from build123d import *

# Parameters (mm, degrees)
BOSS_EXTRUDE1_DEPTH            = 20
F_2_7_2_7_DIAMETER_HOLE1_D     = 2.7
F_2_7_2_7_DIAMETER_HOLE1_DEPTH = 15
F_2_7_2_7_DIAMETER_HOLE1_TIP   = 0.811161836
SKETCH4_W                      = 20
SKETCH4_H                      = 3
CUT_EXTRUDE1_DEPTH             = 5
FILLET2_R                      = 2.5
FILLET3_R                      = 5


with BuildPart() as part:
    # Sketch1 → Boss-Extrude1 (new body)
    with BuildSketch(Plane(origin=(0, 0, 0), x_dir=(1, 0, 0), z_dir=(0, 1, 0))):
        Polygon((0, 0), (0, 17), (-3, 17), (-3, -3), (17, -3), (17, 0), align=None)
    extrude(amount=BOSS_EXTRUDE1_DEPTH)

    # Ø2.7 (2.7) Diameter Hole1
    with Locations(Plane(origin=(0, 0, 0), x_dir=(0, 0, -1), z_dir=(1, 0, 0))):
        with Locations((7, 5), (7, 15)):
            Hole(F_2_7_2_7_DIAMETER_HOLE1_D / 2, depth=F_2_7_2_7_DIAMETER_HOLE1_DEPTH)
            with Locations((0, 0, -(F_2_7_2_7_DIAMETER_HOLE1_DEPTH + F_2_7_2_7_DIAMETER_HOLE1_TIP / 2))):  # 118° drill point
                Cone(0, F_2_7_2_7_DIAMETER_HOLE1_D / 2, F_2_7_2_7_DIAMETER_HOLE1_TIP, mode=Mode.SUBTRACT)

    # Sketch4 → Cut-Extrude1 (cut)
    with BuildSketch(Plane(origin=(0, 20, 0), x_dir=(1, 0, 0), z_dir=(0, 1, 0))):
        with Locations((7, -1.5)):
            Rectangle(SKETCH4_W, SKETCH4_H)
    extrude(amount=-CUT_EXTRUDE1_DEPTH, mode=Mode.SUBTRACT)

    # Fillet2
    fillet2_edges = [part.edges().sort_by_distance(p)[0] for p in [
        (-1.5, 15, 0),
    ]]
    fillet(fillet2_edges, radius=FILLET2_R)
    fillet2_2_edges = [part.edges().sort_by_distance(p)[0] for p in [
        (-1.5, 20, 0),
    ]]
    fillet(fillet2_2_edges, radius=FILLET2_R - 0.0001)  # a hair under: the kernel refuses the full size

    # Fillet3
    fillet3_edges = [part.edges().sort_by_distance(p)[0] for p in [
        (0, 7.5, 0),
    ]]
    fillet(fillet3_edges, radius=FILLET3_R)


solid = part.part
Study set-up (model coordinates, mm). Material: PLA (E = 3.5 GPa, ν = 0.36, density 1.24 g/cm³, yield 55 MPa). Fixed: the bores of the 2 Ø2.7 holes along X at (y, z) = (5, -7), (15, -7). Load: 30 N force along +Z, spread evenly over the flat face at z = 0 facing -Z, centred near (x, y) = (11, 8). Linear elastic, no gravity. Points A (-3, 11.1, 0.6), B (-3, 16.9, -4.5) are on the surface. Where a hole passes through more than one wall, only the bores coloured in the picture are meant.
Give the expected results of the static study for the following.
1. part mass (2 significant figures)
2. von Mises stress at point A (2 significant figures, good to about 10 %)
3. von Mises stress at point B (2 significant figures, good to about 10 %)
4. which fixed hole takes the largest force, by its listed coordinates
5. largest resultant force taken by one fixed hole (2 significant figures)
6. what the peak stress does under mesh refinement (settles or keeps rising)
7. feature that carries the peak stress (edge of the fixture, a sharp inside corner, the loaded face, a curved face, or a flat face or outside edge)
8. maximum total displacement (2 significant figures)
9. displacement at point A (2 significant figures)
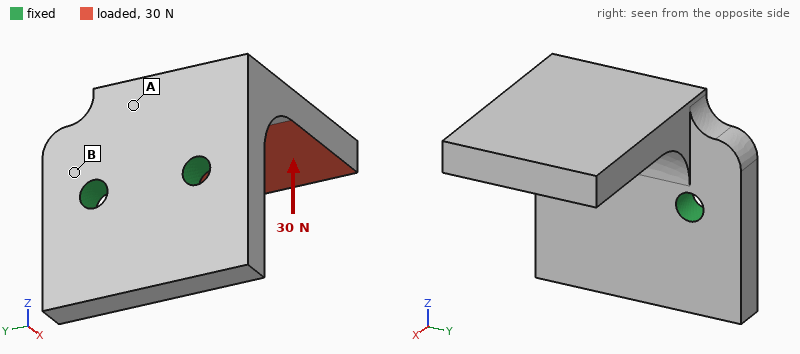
2.4 g
3.2 MPa
7.8 MPa
(5, -7)
22 N
keeps rising
edge of the fixture
0.39 mm
0.060 mm
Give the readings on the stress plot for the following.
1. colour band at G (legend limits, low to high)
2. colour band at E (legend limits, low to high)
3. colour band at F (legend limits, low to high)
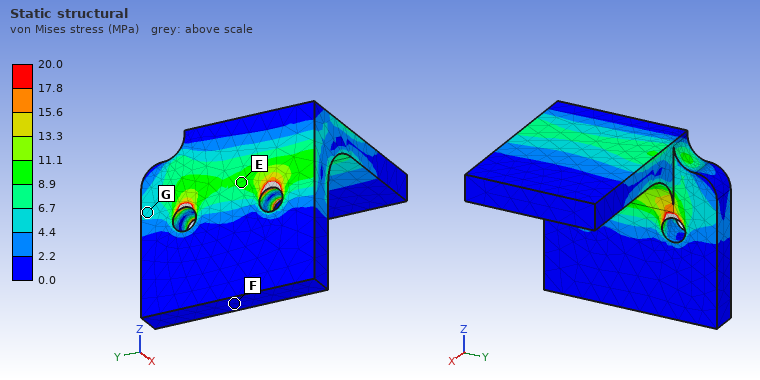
4.4 to 6.7 MPa
8.9 to 11.1 MPa
0.0 to 2.2 MPa
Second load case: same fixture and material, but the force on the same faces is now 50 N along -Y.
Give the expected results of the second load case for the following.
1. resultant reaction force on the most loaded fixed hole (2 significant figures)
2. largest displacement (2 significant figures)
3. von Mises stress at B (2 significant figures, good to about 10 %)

63 N
0.20 mm
5.7 MPa
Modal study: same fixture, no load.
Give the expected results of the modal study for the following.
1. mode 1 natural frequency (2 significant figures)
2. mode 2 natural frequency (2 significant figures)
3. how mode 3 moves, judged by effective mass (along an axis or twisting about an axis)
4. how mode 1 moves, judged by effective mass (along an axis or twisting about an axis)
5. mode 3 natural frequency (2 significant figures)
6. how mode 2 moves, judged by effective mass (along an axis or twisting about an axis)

1900 Hz
3700 Hz
along X
along Z
6100 Hz
along Y
